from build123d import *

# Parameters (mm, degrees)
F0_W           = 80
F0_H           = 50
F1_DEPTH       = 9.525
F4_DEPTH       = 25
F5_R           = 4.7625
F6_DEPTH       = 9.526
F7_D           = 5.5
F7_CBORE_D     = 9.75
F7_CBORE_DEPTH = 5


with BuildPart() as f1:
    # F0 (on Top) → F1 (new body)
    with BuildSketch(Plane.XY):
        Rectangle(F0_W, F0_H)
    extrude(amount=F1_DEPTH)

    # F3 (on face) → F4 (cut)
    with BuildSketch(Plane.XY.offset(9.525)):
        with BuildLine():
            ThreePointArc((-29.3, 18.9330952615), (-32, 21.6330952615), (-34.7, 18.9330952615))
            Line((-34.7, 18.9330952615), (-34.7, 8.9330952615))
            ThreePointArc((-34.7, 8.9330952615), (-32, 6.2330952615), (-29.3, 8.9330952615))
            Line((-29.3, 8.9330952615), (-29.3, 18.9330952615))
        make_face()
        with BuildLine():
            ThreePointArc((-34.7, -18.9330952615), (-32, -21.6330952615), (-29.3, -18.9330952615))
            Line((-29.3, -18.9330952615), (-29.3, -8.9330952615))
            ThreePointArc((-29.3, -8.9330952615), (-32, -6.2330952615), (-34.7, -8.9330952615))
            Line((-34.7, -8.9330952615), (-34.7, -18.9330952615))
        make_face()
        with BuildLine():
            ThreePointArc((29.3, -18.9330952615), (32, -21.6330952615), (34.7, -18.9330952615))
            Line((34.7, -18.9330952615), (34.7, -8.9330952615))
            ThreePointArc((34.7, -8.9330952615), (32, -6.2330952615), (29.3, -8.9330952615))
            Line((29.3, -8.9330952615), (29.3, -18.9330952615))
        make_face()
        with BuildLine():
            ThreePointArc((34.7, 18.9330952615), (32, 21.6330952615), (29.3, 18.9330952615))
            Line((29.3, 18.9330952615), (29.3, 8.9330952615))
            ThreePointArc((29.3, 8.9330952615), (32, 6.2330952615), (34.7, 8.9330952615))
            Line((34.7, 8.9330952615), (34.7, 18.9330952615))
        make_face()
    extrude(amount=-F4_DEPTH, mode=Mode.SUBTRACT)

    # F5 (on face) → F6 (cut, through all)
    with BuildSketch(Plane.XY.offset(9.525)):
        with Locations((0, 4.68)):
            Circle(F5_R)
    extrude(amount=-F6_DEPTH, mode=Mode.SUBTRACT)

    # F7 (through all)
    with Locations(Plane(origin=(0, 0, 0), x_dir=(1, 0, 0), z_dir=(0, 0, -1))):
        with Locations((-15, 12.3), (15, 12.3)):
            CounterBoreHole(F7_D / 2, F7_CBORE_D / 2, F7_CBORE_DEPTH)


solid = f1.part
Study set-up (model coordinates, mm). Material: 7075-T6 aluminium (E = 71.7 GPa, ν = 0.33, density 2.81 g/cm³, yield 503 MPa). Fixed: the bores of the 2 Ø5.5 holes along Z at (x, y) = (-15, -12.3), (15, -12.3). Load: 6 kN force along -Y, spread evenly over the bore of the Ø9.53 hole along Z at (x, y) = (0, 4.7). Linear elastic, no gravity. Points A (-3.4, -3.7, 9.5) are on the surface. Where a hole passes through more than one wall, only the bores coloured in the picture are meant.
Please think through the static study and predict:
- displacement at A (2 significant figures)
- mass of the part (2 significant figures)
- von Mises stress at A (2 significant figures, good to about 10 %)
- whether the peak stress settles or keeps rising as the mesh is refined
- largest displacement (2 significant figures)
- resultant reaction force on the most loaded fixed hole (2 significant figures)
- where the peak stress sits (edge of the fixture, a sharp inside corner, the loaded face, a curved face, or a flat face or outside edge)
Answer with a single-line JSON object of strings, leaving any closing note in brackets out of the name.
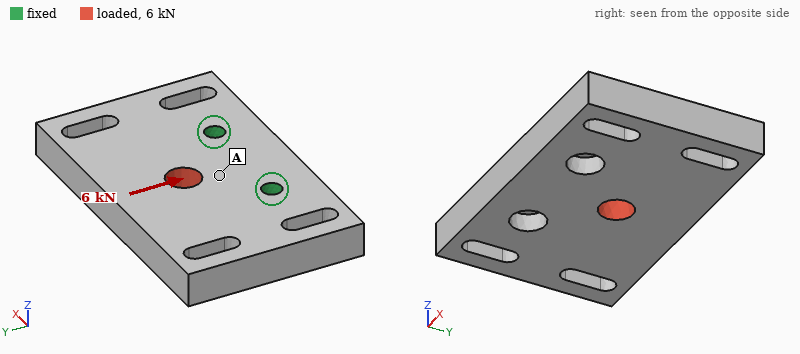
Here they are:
{"displacement at A": "9.8 µm", "mass of the part": "94 g", "von Mises stress at A": "17 MPa", "whether the peak stress settles or keeps rising as the mesh is refined": "keeps rising", "largest displacement": "46 µm", "resultant reaction force on the most loaded fixed hole": "3.1 kN", "where the peak stress sits": "edge of the fixture"}
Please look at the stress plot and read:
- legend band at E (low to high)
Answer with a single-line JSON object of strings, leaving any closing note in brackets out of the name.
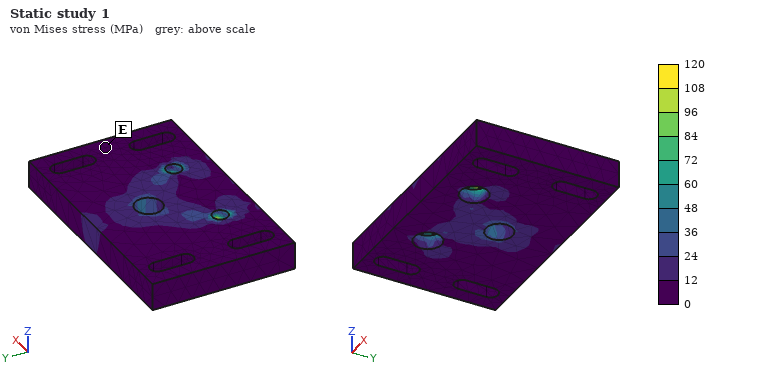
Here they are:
{"legend band at E": "0 to 12 MPa"}
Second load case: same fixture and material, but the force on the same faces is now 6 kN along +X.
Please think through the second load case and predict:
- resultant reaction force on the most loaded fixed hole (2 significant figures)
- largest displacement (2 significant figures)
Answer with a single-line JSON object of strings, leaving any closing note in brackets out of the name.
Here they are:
{"resultant reaction force on the most loaded fixed hole": "4.3 kN", "largest displacement": "31 µm"}
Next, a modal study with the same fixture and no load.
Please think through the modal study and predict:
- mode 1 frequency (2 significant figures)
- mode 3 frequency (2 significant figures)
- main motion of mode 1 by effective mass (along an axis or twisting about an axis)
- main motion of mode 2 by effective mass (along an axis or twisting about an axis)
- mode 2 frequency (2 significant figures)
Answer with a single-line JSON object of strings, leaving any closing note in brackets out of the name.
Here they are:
{"mode 1 frequency": "2800 Hz", "mode 3 frequency": "7900 Hz", "main motion of mode 1 by effective mass": "along Z", "main motion of mode 2 by effective mass": "twisting about Y", "mode 2 frequency": "4600 Hz"}
